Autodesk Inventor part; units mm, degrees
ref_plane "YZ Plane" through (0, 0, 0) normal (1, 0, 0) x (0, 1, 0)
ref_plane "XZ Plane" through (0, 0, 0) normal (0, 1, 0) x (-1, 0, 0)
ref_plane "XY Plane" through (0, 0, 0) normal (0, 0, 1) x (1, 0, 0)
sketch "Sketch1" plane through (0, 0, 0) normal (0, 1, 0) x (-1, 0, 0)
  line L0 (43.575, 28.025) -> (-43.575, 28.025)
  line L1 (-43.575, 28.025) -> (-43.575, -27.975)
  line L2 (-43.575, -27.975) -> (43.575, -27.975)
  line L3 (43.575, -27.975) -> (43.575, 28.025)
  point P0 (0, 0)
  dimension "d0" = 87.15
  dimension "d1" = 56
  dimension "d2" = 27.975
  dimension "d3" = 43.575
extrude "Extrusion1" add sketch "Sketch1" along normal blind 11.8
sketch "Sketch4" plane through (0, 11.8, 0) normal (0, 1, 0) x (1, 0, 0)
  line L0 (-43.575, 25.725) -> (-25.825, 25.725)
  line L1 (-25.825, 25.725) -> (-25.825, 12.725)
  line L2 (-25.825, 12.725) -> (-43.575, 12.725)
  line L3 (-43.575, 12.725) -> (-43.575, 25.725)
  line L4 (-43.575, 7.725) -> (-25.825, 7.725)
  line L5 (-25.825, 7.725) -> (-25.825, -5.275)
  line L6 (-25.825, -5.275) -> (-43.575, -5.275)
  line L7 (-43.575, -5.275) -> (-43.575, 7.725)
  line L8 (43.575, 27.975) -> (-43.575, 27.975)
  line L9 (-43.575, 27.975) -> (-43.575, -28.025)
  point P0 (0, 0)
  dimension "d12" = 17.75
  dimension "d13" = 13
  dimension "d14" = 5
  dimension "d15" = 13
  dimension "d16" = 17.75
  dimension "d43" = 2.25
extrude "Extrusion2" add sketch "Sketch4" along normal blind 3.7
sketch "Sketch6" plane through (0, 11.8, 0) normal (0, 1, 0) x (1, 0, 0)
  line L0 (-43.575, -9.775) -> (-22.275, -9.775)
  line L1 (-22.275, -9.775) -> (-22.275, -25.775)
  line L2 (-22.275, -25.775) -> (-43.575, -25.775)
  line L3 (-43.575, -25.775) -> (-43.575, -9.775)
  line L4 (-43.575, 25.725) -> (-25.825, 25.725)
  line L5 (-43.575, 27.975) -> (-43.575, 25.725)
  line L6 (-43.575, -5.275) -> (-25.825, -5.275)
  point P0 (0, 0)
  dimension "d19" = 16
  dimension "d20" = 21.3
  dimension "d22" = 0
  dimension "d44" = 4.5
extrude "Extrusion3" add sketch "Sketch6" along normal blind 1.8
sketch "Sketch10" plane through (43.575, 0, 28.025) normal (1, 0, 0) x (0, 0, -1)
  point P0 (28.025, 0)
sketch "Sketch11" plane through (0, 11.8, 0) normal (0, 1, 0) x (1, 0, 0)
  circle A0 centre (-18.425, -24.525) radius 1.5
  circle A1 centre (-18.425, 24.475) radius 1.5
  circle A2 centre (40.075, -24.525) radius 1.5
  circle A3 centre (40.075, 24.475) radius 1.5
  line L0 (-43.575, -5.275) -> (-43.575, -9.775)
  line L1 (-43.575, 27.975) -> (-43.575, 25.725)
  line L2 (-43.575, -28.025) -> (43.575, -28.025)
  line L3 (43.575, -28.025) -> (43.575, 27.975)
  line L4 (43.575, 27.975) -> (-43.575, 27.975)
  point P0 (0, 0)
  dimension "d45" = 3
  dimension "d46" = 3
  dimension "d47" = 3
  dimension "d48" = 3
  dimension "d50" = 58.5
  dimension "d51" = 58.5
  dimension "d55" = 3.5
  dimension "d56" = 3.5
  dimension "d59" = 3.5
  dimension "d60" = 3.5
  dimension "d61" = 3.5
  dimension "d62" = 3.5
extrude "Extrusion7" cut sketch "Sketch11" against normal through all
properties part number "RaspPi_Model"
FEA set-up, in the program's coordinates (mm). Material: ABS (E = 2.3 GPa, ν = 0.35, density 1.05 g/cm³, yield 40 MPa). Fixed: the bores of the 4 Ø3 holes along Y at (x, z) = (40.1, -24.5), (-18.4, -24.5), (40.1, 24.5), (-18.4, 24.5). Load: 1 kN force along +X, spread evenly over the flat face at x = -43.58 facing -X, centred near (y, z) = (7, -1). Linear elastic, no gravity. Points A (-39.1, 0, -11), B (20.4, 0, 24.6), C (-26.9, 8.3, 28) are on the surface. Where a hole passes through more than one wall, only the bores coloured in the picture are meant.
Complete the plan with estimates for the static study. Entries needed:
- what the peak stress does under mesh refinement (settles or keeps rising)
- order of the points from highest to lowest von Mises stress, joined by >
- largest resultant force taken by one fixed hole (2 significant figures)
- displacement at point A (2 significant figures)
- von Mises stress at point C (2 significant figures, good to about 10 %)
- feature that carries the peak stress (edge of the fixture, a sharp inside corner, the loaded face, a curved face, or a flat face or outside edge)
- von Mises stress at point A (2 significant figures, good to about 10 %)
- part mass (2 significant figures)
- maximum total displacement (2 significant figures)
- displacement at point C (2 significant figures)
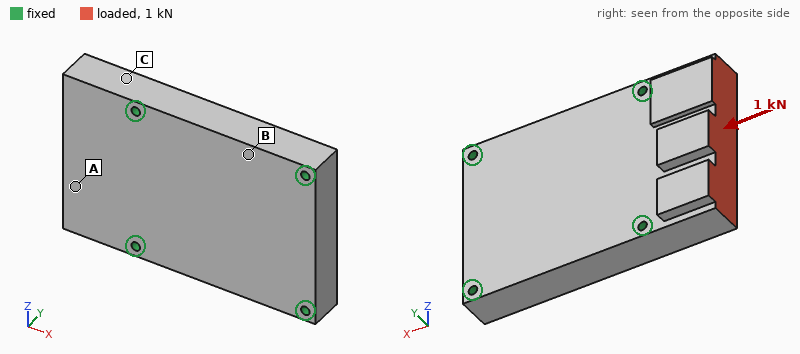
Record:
keeps rising
C > A > B
430 N
25 µm
2.3 MPa
edge of the fixture
1.1 MPa
63 g
48 µm
11 µm
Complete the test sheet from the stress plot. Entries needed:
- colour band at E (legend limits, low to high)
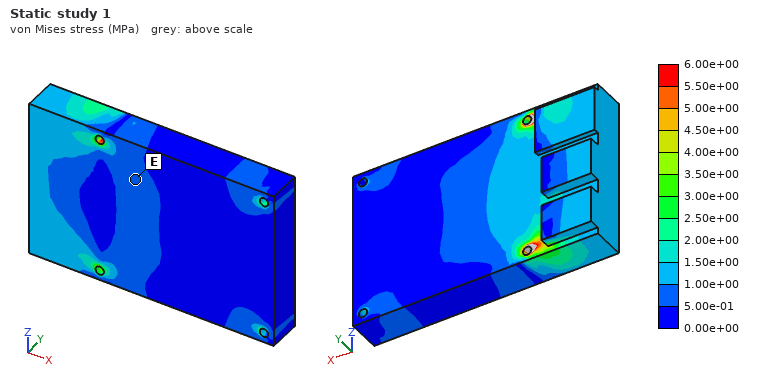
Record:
5.00e-01 to 1.00e+00 MPa
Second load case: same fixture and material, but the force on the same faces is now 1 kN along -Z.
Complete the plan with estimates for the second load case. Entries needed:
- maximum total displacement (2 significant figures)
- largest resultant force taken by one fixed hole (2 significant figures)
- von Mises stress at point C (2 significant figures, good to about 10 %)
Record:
94 µm
700 N
3.0 MPa
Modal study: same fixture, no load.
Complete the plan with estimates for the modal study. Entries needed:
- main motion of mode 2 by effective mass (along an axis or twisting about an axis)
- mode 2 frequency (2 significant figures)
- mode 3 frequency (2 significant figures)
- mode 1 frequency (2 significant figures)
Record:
along Y
3000 Hz
4500 Hz
2400 Hz
